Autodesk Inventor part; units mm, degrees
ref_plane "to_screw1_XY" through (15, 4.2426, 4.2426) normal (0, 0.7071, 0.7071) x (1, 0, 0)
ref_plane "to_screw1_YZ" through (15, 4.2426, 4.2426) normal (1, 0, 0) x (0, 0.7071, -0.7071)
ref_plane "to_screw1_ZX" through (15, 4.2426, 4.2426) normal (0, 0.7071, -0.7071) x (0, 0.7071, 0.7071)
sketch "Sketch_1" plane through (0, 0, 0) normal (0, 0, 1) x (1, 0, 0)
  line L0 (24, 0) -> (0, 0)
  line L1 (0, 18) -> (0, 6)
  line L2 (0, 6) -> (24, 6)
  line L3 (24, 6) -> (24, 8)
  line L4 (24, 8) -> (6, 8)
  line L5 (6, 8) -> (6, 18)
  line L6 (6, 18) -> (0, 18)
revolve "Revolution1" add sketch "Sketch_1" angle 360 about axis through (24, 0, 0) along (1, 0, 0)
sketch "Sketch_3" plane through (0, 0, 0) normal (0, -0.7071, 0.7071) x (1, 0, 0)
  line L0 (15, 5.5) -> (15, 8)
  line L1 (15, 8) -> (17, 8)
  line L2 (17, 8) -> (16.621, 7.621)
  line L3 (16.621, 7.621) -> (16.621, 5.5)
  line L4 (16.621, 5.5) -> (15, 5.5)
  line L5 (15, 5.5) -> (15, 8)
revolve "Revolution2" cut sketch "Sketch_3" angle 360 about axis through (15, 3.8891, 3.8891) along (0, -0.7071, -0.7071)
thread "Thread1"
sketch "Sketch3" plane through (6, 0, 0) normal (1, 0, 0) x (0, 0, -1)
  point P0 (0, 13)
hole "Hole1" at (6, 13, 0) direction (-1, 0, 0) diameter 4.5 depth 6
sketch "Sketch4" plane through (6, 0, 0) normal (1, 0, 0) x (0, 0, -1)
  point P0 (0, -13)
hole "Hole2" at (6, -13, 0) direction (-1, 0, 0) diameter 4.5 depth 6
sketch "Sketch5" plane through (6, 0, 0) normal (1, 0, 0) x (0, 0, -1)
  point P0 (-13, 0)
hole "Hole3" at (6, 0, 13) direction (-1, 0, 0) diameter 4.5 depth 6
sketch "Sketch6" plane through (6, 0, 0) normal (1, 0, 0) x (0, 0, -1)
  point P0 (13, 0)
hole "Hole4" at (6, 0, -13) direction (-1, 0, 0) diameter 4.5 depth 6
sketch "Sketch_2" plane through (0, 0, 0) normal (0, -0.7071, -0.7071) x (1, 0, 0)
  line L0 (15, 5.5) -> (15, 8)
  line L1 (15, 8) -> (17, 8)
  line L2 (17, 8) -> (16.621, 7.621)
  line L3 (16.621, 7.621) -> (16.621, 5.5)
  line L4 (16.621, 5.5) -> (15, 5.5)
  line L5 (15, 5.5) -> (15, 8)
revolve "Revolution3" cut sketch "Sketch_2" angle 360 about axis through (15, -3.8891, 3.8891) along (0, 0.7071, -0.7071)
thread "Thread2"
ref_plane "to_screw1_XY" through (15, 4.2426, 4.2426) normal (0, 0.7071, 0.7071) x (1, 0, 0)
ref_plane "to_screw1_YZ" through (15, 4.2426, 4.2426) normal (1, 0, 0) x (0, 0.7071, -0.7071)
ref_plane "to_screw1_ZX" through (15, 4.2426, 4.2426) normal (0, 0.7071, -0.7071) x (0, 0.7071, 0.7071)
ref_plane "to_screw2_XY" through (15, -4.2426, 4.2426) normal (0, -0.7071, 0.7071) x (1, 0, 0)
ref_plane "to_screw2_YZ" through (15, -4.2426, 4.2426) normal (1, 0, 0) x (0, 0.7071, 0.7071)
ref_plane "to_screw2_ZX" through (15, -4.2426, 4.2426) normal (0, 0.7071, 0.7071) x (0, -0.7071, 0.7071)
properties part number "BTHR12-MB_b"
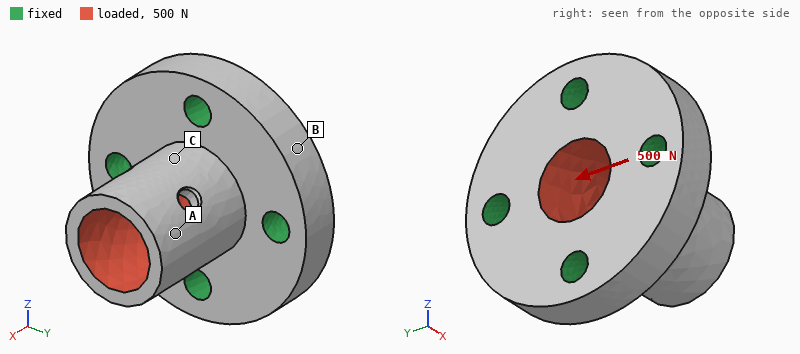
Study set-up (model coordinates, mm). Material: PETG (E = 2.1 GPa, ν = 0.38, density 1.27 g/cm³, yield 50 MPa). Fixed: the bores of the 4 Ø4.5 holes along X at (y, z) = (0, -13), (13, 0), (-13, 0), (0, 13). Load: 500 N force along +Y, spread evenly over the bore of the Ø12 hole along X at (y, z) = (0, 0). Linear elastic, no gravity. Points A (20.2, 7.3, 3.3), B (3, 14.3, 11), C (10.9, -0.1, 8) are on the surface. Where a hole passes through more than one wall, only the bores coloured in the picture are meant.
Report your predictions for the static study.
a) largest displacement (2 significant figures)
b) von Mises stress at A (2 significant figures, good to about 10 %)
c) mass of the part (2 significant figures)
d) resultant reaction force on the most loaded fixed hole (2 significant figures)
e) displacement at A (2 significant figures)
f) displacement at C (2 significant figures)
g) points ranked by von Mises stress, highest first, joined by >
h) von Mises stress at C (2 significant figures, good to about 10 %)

0.25 mm
3.2 MPa
8.4 g
250 N
0.21 mm
0.072 mm
C > A > B
6.7 MPa
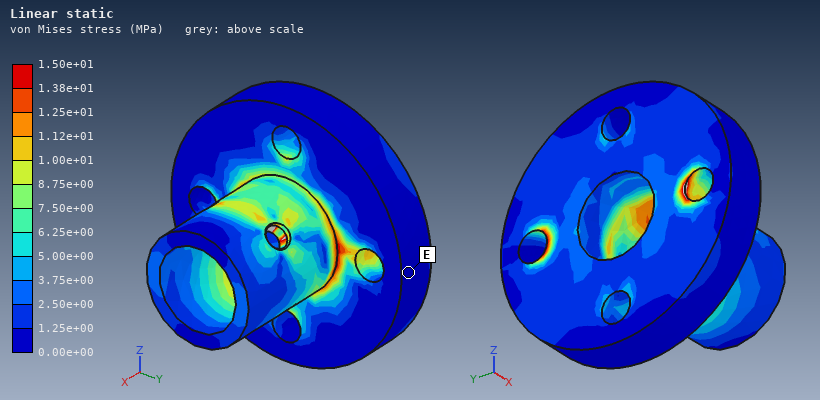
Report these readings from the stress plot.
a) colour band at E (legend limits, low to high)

0.00e+00 to 1.25e+00 MPa
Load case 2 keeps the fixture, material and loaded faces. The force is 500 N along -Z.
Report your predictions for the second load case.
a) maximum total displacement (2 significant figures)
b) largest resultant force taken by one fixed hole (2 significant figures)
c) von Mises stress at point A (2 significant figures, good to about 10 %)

0.25 mm
250 N
2.3 MPa
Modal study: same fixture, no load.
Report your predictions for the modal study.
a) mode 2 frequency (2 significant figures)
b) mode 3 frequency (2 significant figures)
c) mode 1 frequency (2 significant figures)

5100 Hz
7400 Hz
5100 Hz
